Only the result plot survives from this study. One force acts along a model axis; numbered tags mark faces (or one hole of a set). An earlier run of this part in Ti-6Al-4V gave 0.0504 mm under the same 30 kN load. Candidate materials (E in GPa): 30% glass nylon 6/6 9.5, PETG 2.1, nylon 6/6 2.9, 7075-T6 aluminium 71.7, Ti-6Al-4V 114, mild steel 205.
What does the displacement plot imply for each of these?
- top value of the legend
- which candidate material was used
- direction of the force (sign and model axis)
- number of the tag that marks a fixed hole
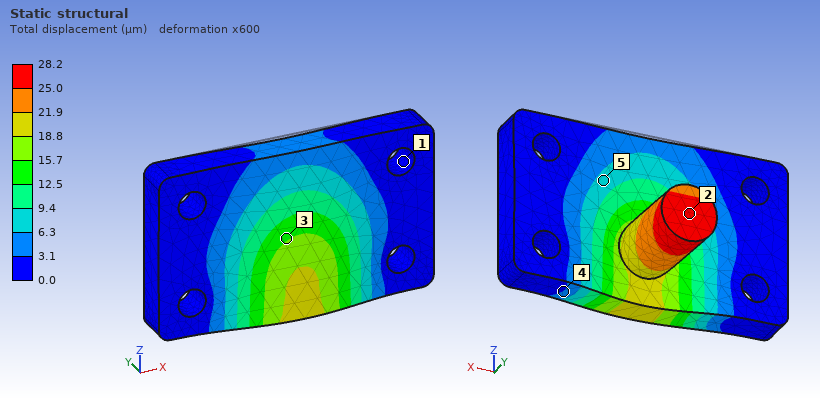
28.2 µm
mild steel
-Y
1
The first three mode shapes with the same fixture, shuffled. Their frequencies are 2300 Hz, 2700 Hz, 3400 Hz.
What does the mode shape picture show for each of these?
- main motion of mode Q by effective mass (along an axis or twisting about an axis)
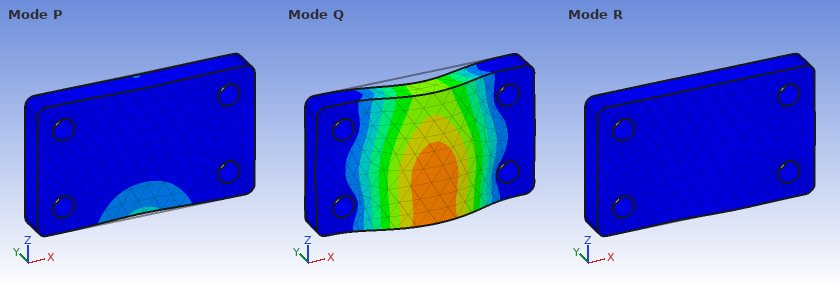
along Y
